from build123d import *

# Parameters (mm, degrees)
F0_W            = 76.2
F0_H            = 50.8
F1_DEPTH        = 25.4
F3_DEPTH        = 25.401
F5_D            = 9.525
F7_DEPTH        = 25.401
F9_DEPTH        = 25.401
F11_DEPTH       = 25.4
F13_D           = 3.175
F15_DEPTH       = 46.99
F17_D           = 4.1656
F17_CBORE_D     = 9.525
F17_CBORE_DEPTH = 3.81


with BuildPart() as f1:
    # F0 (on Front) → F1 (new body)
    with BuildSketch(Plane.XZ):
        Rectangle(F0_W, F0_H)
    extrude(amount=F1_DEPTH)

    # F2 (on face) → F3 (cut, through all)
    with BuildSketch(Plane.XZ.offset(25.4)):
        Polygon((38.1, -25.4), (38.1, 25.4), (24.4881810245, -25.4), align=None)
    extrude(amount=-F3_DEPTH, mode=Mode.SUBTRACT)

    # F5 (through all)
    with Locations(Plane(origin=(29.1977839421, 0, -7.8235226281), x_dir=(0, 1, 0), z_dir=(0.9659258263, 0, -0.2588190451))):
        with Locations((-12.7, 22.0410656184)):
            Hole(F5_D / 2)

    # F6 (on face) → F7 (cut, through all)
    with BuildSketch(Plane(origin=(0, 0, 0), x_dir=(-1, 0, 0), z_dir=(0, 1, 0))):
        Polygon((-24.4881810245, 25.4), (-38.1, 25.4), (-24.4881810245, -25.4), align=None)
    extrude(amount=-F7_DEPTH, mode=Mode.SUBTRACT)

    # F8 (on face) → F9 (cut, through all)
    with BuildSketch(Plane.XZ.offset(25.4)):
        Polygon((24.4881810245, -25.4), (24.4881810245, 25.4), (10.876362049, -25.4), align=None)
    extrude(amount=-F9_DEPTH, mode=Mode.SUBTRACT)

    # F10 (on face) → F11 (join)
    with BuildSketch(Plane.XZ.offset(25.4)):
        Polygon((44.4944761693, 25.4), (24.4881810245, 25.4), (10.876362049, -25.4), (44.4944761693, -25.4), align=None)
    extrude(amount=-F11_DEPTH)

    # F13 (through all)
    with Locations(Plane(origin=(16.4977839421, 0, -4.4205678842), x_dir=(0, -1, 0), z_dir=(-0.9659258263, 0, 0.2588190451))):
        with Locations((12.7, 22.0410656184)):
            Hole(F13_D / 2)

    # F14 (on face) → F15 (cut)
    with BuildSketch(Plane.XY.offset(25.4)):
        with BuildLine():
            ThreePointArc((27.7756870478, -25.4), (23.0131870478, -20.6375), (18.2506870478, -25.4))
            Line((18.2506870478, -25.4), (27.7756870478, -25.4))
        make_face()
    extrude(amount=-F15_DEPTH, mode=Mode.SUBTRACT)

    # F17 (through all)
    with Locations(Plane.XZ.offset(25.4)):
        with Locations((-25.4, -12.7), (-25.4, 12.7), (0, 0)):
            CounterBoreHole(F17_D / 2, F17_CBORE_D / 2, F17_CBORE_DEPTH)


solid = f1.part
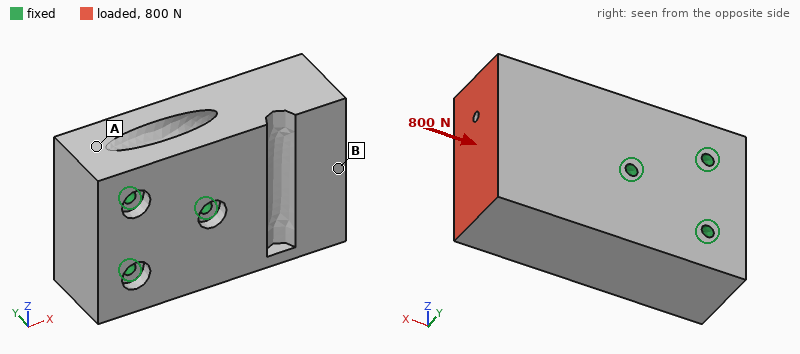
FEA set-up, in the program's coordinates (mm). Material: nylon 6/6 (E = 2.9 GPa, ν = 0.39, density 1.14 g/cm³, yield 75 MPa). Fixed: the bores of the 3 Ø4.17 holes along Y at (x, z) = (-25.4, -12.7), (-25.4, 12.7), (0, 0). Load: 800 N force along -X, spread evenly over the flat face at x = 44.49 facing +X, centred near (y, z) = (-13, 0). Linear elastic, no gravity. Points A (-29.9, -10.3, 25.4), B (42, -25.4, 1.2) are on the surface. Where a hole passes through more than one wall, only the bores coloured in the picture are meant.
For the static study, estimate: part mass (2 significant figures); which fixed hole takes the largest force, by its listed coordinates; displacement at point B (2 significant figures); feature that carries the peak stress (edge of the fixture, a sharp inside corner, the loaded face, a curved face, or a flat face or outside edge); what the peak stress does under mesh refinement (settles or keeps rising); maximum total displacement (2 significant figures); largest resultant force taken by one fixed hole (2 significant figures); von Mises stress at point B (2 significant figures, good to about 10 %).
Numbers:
110 g
(0, 0)
19 µm
edge of the fixture
keeps rising
22 µm
450 N
0.66 MPa
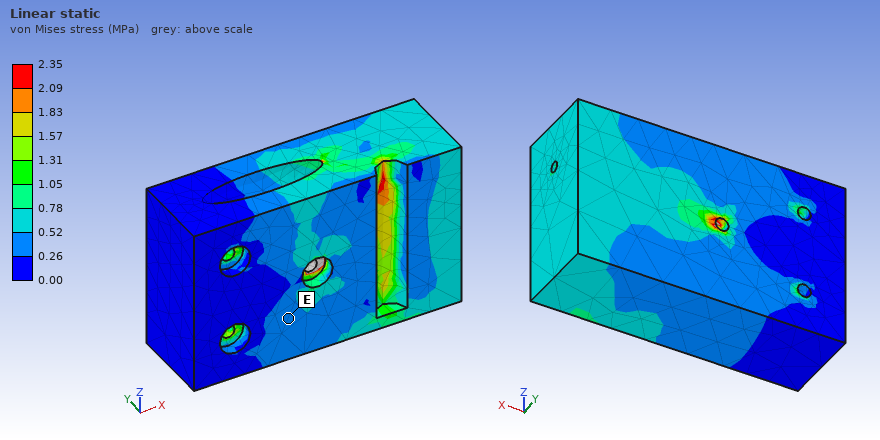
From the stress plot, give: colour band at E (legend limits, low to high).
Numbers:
0.26 to 0.52 MPa
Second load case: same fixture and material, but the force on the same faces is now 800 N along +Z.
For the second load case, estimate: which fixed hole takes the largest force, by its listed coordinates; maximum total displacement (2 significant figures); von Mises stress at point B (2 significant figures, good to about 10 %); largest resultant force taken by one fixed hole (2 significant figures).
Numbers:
(0, 0)
0.16 mm
1.4 MPa
1.4 kN
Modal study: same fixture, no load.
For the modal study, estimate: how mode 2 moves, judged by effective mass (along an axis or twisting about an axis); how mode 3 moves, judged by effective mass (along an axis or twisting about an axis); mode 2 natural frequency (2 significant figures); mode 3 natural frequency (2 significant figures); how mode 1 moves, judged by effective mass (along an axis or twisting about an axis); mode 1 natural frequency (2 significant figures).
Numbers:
along Z
twisting about X
2500 Hz
3000 Hz
along Y
1900 Hz
